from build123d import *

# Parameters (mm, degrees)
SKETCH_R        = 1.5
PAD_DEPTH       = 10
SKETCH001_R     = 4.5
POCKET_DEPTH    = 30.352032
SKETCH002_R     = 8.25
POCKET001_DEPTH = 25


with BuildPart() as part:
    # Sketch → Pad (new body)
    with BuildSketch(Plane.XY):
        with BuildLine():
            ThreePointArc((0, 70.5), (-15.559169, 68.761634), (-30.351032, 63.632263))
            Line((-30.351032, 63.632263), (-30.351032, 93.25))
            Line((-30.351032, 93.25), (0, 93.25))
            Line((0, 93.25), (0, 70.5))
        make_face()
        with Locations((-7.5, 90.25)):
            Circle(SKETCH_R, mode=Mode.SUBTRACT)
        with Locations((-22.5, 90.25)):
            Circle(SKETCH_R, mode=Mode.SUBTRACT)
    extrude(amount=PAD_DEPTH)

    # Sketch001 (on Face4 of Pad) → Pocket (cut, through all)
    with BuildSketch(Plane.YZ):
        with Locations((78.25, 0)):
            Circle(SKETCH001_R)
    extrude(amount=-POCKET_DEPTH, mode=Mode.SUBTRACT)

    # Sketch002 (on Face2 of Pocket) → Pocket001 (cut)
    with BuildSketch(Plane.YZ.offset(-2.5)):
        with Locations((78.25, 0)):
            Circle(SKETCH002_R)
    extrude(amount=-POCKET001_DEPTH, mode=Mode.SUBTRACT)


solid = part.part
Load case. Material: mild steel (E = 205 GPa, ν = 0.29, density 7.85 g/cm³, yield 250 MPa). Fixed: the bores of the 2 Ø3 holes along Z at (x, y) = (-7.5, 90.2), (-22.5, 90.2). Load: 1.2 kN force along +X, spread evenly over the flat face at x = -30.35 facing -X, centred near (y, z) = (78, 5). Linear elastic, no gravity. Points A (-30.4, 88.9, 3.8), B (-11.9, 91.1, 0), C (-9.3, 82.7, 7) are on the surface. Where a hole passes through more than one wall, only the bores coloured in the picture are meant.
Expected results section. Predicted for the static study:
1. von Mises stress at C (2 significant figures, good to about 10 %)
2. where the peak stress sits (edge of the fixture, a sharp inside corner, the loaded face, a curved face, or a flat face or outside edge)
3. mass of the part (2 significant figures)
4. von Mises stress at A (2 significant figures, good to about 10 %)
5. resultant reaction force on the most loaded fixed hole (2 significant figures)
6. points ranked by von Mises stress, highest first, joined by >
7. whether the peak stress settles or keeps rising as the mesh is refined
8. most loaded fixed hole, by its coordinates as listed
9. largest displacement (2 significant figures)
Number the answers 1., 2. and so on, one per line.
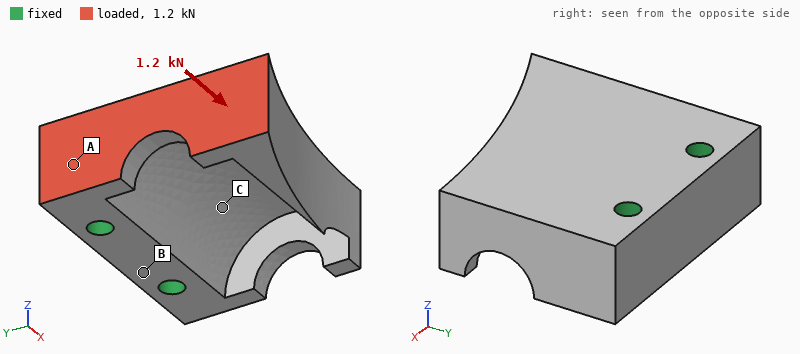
1. 28 MPa
2. edge of the fixture
3. 36 g
4. 13 MPa
5. 1.1 kN
6. C > A > B
7. keeps rising
8. (-22.5, 90.2)
9. 13 µm
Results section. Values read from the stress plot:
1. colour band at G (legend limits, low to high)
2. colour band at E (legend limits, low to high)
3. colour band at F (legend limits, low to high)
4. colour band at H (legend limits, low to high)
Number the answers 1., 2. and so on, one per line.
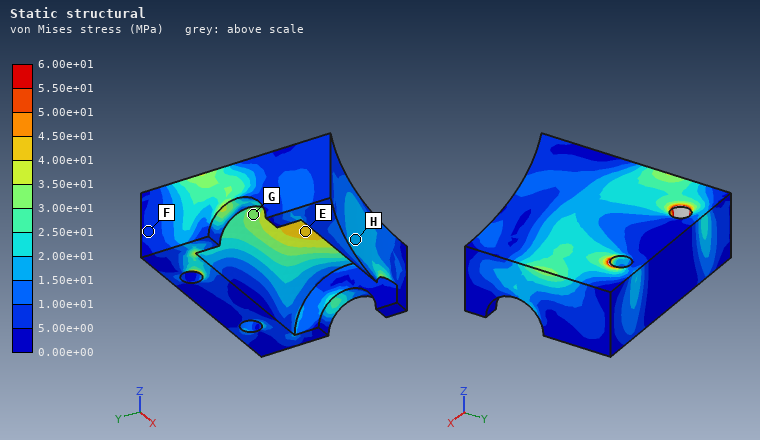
1. 3.00e+01 to 3.50e+01 MPa
2. 4.00e+01 to 4.50e+01 MPa
3. 5.00e+00 to 1.00e+01 MPa
4. 1.50e+01 to 2.00e+01 MPa
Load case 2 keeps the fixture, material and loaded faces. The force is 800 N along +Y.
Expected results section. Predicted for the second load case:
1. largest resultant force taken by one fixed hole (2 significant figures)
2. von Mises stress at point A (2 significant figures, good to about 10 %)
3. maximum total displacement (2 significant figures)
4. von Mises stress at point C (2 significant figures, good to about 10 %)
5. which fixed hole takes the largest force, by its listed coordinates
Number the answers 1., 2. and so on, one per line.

1. 1.1 kN
2. 9.9 MPa
3. 11 µm
4. 9.4 MPa
5. (-22.5, 90.2)
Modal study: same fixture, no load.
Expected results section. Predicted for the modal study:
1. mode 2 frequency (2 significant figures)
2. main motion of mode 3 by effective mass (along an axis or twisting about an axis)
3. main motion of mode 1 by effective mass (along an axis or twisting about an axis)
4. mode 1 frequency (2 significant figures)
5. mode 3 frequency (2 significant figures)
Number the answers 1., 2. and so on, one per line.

1. 12 kHz
2. along X
3. along Z
4. 6400 Hz
5. 19 kHz
